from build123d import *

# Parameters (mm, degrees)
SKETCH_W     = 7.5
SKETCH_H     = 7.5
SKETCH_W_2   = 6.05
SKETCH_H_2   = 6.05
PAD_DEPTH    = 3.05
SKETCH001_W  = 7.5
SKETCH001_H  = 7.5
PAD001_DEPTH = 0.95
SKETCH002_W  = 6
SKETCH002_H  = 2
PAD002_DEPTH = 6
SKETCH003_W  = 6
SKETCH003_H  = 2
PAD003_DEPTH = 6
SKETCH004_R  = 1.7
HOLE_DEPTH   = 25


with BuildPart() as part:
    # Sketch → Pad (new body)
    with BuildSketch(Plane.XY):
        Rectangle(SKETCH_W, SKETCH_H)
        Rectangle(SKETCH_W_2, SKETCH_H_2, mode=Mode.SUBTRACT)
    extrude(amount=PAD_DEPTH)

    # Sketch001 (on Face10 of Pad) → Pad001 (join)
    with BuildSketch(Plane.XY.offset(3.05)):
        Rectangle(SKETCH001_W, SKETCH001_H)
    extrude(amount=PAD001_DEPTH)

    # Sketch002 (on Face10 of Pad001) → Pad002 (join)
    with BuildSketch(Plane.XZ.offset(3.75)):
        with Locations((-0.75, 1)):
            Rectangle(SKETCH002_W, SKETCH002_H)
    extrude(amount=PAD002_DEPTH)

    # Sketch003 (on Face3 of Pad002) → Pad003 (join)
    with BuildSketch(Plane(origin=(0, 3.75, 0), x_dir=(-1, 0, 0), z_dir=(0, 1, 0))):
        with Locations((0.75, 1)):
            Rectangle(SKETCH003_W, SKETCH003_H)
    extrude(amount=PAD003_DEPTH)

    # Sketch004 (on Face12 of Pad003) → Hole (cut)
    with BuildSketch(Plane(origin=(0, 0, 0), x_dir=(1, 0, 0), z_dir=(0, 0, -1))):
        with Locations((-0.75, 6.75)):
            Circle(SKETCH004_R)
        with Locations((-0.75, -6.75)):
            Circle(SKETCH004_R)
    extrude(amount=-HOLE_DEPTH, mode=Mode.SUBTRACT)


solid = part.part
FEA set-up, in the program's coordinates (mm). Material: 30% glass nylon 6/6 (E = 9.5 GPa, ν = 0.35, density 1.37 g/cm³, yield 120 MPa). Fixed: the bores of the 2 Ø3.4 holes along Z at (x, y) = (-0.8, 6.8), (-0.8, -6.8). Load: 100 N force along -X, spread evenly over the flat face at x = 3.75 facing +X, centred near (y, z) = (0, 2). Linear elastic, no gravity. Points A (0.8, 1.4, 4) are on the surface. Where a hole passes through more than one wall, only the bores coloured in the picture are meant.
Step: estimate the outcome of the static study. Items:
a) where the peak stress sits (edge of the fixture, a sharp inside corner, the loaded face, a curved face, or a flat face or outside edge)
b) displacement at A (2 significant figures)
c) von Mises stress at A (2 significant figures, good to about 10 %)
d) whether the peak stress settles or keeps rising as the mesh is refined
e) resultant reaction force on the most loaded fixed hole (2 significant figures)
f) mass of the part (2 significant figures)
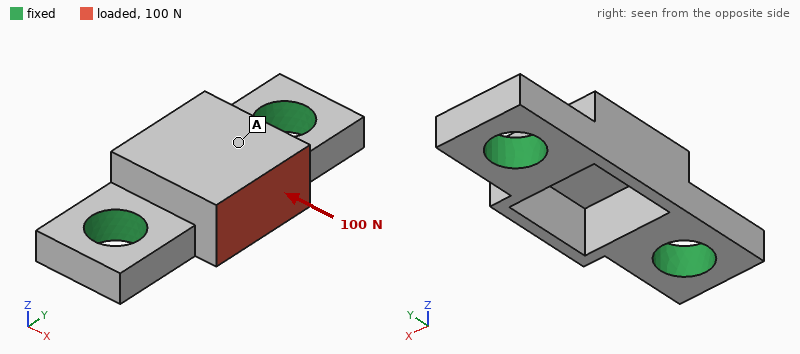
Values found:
a sharp inside corner
15 µm
8.2 MPa
keeps rising
51 N
0.30 g
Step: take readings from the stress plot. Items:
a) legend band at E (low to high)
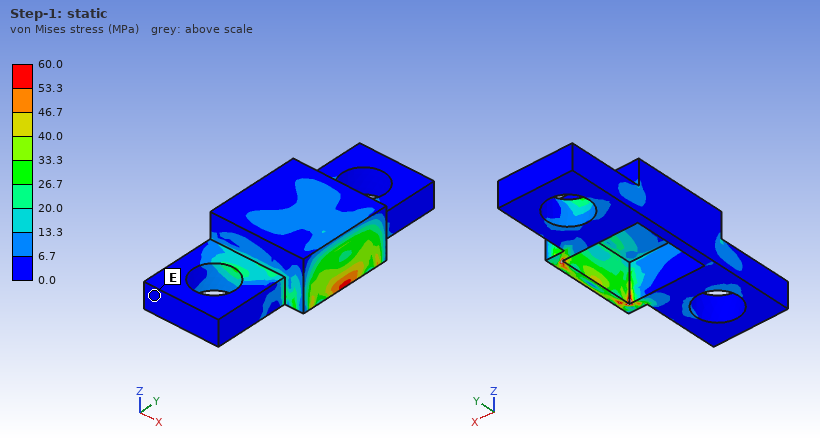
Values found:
0.0 to 6.7 MPa
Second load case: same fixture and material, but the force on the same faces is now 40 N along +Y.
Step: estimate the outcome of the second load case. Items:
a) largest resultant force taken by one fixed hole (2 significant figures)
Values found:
24 N
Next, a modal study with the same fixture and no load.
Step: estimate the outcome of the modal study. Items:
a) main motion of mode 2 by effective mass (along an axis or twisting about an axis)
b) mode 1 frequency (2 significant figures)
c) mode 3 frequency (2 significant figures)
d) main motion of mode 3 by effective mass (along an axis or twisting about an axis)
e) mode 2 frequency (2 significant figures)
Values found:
along Y
26 kHz
41 kHz
along Z
40 kHz
